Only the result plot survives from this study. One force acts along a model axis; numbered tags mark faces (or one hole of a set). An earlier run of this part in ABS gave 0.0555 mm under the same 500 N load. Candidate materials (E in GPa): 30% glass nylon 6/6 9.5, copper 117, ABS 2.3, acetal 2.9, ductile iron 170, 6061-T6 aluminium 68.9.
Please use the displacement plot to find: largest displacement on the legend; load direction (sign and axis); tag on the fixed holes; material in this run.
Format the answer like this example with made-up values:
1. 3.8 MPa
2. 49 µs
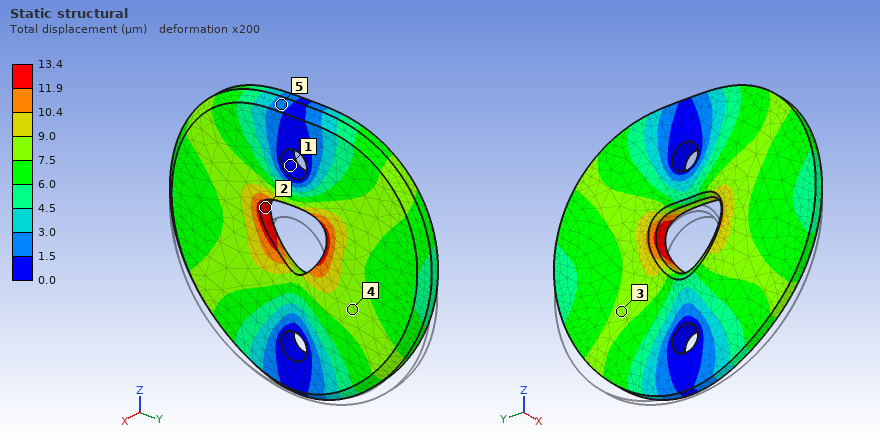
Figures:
1. 13.4 µm
2. +Z
3. 1
4. 30% glass nylon 6/6
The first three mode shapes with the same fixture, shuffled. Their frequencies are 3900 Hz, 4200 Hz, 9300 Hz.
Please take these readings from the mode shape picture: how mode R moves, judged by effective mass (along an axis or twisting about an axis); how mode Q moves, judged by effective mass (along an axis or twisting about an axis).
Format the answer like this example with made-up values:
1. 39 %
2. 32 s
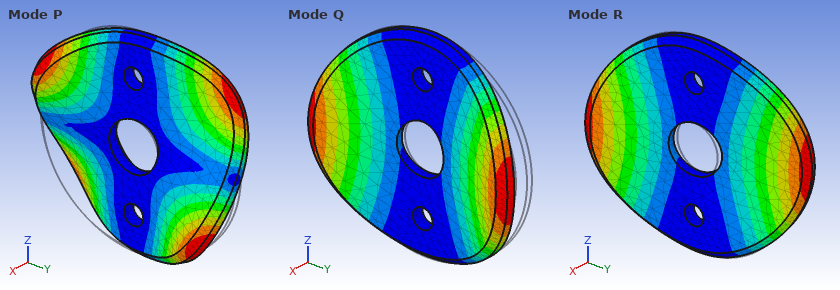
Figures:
1. twisting about Z
2. along X
